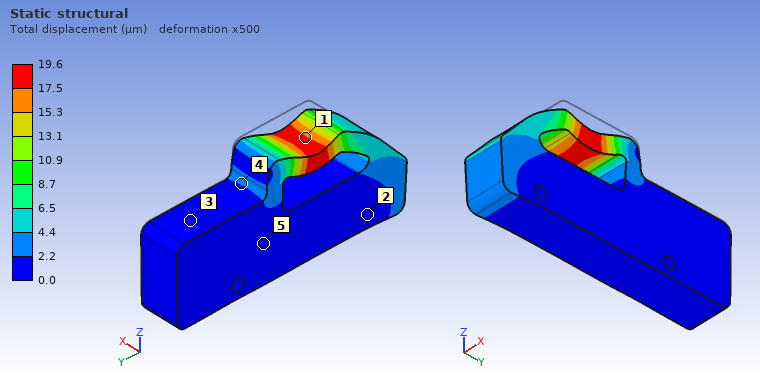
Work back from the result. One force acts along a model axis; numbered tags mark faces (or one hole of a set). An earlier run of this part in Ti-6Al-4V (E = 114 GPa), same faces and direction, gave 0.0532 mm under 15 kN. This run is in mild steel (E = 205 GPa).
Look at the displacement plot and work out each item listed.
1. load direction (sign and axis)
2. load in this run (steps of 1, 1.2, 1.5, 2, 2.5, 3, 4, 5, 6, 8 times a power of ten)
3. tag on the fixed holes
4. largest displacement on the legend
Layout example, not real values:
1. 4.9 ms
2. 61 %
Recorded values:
1. -Z
2. 10 kN
3. 2
4. 19.6 µm
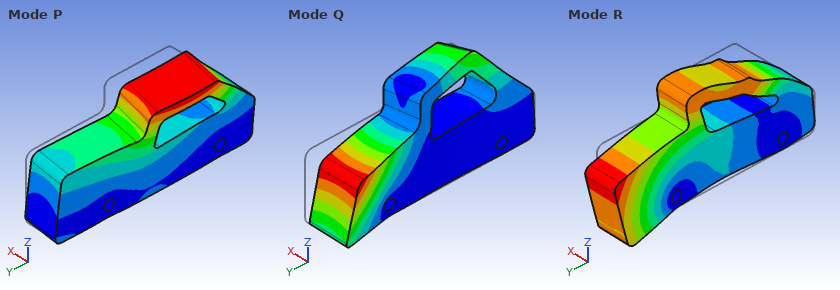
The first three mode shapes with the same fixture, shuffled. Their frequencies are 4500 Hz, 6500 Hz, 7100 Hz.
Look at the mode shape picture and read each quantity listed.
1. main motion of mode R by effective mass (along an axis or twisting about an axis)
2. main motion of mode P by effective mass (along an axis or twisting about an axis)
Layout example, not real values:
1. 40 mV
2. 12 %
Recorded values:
1. along Y
2. along X
